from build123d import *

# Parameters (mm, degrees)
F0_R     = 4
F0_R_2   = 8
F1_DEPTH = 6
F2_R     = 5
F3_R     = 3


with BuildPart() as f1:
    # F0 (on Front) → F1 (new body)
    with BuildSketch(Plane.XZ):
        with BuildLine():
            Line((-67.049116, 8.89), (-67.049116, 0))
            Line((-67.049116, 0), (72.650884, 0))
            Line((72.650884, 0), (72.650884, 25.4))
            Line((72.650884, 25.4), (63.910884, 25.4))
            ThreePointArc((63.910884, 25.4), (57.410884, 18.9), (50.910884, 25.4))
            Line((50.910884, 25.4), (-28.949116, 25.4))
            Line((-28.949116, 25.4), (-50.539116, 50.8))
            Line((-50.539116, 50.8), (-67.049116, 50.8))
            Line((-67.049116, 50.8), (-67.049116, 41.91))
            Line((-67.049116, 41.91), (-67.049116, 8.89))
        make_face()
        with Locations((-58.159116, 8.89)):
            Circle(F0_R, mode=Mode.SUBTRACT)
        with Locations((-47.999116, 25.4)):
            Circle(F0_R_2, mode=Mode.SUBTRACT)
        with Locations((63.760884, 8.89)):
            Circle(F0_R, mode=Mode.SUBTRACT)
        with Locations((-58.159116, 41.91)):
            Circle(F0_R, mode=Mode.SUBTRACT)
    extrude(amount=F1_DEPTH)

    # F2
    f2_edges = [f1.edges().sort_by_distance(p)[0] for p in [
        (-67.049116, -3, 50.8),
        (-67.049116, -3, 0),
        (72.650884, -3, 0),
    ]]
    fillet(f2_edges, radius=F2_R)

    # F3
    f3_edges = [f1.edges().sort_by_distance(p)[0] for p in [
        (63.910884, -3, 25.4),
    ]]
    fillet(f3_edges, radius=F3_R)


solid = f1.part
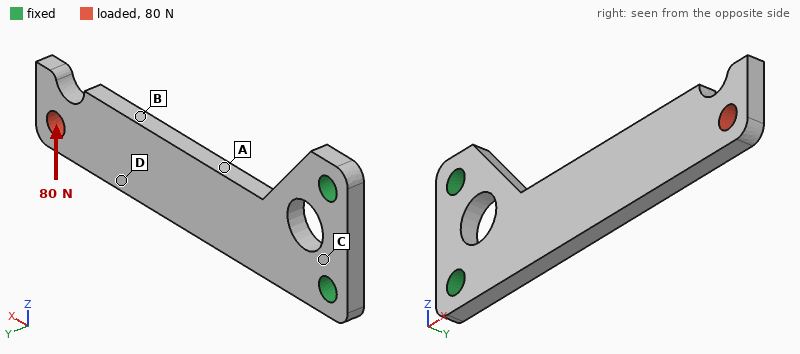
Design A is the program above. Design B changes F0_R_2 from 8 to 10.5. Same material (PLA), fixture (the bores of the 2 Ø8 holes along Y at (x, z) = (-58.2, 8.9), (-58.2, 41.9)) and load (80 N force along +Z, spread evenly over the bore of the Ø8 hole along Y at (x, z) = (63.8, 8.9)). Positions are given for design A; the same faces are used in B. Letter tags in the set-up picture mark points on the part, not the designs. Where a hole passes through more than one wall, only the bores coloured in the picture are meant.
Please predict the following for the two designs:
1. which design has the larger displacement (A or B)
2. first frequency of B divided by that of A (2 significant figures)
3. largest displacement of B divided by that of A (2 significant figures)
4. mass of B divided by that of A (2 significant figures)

B
0.94
1.1
0.96
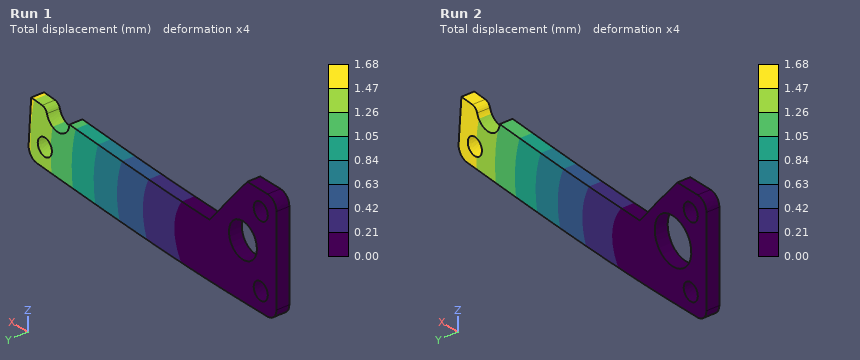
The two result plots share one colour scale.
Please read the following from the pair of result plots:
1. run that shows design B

Run 2
